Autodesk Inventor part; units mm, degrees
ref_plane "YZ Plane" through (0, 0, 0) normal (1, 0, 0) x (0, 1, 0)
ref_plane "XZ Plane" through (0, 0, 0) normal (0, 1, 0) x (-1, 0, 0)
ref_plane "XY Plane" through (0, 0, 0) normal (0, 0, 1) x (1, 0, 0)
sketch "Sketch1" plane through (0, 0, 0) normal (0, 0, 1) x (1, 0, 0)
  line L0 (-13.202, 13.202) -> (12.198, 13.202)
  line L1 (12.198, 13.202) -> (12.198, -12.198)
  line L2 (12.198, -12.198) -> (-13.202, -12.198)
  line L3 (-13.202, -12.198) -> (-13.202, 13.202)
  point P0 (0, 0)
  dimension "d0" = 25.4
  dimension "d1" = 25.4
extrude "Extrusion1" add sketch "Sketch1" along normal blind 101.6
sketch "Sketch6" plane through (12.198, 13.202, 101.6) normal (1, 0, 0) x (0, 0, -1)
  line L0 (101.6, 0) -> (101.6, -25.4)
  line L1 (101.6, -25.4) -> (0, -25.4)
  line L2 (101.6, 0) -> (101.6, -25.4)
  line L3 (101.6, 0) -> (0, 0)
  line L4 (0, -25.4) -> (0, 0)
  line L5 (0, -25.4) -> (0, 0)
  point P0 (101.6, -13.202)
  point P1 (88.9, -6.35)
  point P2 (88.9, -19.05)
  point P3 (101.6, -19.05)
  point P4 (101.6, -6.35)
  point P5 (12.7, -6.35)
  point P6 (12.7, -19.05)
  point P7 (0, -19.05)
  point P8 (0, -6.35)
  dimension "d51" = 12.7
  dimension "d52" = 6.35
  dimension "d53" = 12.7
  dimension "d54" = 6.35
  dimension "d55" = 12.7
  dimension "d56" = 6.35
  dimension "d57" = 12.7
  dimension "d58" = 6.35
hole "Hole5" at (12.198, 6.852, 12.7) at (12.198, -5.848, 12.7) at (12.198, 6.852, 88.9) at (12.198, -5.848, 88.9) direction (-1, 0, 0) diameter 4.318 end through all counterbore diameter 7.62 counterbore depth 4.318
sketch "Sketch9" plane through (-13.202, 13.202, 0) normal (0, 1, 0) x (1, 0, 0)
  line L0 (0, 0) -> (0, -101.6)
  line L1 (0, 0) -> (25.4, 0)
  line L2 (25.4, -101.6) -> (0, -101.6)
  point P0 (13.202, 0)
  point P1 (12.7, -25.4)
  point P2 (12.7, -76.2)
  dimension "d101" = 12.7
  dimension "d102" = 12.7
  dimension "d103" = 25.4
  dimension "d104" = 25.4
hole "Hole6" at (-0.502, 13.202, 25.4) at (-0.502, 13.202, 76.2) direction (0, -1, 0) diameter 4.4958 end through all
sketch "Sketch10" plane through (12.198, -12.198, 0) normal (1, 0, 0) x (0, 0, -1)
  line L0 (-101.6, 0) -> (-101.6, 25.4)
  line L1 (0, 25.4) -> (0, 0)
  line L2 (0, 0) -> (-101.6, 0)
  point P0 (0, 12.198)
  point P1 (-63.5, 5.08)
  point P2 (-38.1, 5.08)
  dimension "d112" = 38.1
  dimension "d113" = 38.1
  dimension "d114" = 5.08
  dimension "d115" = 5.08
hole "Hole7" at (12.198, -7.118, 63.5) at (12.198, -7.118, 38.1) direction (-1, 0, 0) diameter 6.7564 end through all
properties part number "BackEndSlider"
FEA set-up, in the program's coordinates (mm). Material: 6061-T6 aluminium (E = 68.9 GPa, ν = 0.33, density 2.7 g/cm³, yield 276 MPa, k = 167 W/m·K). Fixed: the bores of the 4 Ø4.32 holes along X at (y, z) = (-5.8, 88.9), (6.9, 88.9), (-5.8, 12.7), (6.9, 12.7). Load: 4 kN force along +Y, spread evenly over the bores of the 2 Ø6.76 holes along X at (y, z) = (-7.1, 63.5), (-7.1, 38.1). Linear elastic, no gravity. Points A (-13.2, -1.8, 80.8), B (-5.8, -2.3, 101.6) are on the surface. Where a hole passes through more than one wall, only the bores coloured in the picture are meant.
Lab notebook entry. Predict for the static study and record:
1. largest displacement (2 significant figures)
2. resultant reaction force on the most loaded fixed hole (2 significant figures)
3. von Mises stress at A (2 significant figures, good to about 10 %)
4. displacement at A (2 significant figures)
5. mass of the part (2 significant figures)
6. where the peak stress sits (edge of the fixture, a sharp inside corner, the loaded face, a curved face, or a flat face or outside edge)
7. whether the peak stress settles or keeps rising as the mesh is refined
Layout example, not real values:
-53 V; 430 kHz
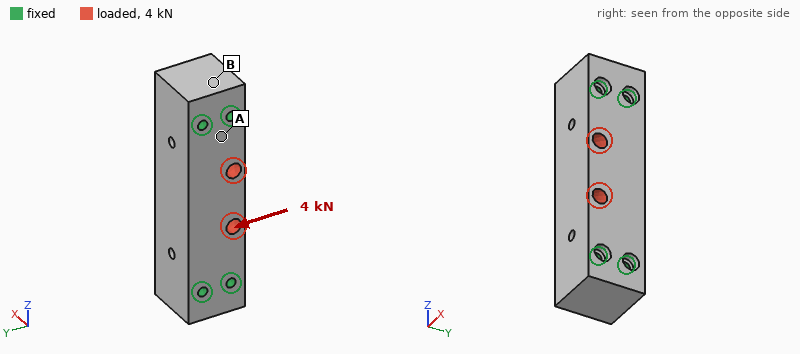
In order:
8.2 µm; 2.2 kN; 9.5 MPa; 1.5 µm; 160 g; edge of the fixture; keeps rising
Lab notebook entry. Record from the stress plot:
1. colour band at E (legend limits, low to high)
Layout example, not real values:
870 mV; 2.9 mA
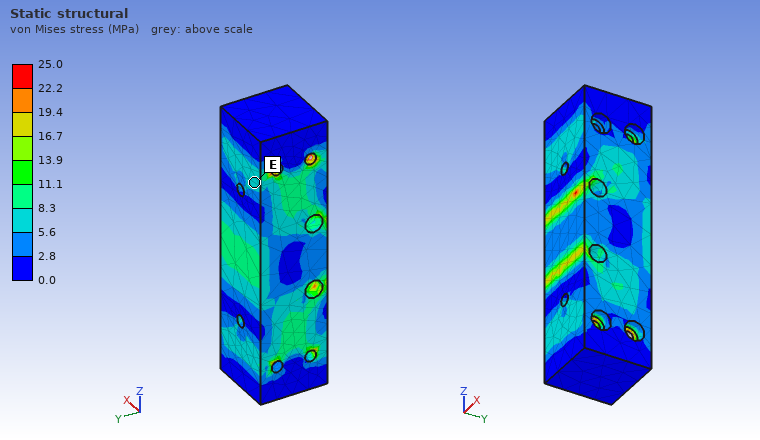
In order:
5.6 to 8.3 MPa
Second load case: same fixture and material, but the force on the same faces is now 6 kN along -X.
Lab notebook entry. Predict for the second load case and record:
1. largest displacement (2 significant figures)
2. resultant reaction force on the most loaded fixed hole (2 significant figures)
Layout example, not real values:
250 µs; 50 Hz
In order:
20 µm; 2.3 kN
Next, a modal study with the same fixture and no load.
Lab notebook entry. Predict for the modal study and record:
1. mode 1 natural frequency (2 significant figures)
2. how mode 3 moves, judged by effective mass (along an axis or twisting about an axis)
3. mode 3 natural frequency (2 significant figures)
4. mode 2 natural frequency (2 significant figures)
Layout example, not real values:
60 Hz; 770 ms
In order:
13 kHz; twisting about Z; 18 kHz; 14 kHz
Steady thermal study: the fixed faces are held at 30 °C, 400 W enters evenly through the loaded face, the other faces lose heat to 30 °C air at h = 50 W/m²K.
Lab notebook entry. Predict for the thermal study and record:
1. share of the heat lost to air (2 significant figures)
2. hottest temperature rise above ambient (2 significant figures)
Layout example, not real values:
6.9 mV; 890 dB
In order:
3.5 %; 66 K
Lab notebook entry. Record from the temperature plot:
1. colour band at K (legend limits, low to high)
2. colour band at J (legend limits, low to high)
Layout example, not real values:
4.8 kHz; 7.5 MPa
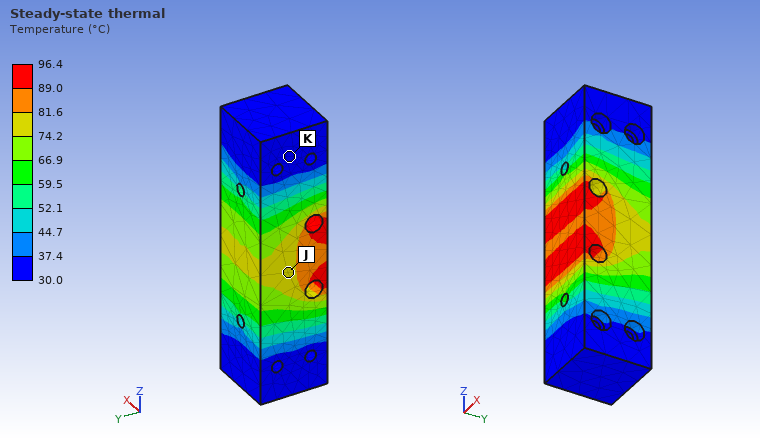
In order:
30.0 to 37.4 °C; 74.2 to 81.6 °C
